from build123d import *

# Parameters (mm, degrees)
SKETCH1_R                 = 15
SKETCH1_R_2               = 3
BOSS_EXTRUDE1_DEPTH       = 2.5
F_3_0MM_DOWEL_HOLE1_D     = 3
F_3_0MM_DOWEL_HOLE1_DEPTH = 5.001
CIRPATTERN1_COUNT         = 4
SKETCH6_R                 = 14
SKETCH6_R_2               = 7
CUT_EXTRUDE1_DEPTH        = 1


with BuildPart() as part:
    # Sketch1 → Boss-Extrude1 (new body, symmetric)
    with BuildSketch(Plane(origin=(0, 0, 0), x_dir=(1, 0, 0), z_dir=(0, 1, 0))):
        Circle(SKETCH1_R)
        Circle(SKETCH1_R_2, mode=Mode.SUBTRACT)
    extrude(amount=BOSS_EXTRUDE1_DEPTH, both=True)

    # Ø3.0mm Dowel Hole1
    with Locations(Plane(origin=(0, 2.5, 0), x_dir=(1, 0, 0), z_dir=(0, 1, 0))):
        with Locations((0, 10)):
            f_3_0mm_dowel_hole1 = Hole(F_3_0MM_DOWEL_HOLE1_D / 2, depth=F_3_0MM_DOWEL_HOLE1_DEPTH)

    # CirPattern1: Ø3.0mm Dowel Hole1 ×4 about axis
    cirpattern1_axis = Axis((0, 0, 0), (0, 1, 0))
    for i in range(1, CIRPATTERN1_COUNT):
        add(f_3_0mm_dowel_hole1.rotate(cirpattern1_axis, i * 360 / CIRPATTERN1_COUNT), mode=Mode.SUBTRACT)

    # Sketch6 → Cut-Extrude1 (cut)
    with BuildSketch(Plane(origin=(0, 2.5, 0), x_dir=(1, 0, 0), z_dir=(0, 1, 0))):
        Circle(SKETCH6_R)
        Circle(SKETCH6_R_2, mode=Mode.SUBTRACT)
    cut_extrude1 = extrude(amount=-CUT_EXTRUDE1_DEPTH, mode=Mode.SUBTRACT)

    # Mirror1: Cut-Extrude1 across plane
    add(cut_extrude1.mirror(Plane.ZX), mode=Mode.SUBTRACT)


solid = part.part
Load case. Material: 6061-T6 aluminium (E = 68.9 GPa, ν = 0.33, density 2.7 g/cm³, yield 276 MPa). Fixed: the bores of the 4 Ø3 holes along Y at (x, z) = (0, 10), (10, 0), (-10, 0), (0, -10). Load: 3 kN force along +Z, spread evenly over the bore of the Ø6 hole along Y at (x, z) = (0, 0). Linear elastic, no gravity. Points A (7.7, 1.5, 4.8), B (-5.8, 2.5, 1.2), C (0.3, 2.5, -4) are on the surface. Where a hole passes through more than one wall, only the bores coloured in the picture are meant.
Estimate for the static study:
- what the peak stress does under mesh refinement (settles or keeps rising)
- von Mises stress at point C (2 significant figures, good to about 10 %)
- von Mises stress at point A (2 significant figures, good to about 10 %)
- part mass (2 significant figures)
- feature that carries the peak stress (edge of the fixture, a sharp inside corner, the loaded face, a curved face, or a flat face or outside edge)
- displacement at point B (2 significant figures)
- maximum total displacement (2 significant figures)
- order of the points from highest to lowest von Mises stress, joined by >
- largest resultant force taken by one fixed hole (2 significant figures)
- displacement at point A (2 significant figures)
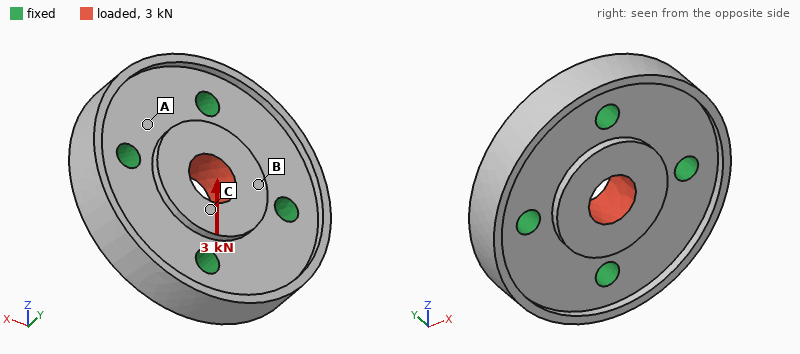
keeps rising
34 MPa
12 MPa
6.4 g
edge of the fixture
2.2 µm
4.4 µm
C > A > B
990 N
1.5 µm
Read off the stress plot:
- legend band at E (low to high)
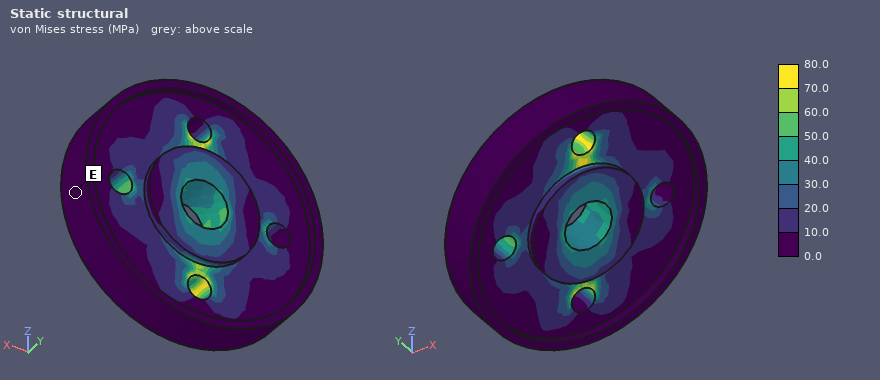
0.0 to 10.0 MPa
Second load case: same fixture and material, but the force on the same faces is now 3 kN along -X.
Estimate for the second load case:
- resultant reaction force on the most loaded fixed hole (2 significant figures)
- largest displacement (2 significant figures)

990 N
4.4 µm
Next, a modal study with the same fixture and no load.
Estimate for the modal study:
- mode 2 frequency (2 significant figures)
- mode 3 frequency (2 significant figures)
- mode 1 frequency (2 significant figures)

40 kHz
40 kHz
37 kHz
